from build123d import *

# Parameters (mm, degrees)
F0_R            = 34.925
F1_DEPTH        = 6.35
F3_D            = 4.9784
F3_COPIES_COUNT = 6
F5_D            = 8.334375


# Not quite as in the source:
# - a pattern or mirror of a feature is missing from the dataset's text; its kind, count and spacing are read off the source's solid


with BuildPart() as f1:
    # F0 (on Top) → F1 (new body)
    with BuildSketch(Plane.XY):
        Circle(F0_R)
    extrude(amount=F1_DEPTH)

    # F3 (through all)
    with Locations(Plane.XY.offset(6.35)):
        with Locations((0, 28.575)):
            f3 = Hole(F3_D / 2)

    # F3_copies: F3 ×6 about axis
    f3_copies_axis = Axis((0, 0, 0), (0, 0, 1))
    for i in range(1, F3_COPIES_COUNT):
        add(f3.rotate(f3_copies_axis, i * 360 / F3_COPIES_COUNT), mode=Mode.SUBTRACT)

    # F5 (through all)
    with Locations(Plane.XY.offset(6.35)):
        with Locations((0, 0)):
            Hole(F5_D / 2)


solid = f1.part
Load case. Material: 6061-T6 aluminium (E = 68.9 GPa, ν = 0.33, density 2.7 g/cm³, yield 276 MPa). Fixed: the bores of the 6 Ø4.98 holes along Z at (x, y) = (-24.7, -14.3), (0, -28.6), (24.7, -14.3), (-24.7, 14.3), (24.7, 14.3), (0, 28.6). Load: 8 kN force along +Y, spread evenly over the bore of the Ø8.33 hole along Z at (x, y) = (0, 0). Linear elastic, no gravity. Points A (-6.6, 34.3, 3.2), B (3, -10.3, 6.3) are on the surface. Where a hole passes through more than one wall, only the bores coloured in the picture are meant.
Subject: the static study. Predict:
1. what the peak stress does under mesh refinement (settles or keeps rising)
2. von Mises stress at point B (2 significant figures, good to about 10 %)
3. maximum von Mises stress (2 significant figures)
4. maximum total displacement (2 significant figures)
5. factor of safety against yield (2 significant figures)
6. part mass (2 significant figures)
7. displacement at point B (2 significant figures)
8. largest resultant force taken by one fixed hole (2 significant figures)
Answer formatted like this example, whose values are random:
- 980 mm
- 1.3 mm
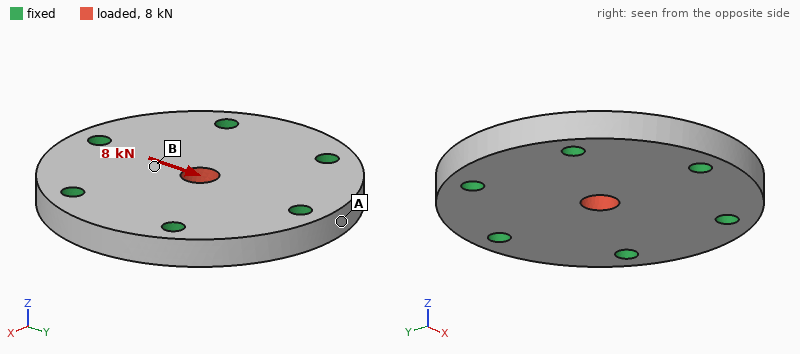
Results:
- settles
- 31 MPa
- 85 MPa
- 10 µm
- 3.2
- 63 g
- 6.4 µm
- 2.1 kN
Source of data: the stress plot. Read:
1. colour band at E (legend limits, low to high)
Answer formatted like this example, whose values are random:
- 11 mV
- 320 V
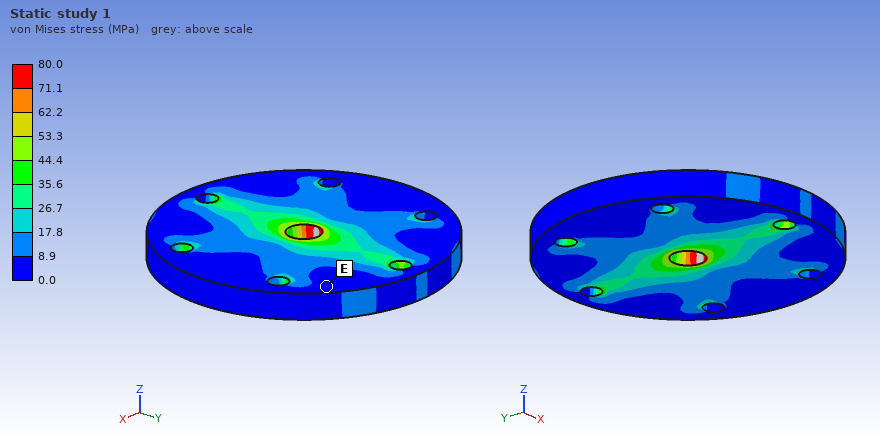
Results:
- 0.0 to 8.9 MPa
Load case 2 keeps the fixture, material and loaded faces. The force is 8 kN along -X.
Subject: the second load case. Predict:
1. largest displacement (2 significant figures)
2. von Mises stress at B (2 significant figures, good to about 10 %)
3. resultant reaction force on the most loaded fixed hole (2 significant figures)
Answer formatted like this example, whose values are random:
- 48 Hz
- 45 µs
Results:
- 10 µm
- 15 MPa
- 1.8 kN
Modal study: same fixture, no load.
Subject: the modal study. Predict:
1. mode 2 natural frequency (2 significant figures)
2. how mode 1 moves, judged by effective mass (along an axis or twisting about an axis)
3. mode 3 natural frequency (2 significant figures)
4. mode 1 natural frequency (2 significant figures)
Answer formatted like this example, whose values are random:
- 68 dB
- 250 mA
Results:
- 28 kHz
- along Z
- 28 kHz
- 16 kHz
